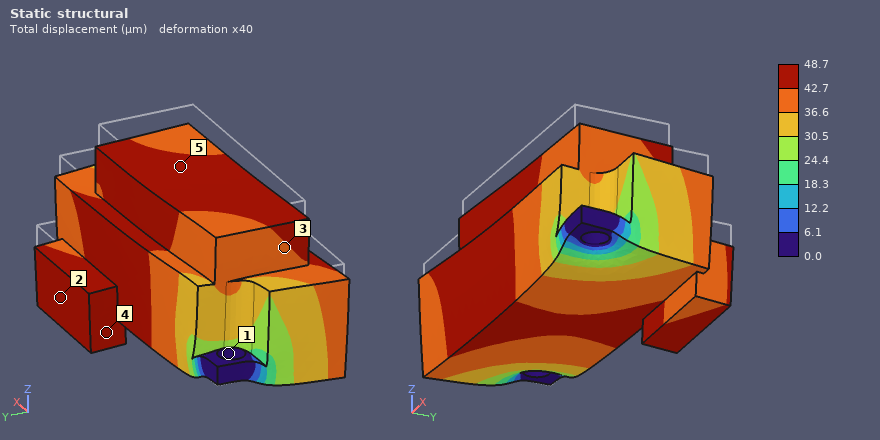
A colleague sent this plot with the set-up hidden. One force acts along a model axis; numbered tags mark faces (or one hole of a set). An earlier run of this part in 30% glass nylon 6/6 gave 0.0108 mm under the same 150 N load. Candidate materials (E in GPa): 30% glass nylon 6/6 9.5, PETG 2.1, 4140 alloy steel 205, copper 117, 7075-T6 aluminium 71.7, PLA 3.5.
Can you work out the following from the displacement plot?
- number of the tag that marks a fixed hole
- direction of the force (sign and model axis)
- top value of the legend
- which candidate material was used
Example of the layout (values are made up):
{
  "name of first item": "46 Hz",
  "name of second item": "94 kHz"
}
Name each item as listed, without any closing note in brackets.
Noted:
{
  "number of the tag that marks a fixed hole": "1",
  "direction of the force": "-Z",
  "top value of the legend": "48.7 µm",
  "which candidate material was used": "PETG"
}
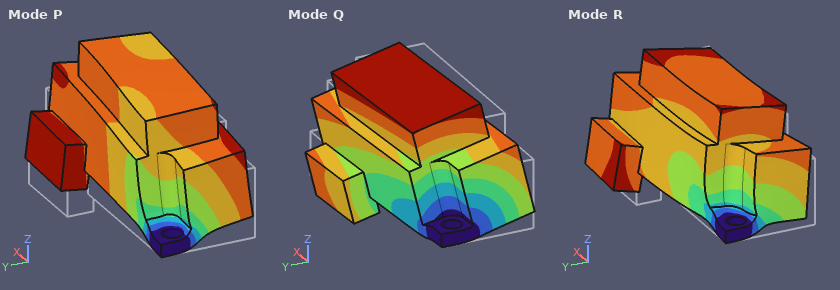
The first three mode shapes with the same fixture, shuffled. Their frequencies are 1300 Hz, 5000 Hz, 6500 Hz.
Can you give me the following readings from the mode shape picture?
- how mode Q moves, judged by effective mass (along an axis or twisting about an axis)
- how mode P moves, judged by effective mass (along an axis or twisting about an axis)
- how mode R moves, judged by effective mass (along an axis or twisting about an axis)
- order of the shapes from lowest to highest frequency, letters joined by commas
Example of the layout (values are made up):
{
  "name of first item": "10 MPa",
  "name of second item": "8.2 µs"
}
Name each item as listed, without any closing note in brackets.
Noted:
{
  "how mode Q moves, judged by effective mass": "along Y",
  "how mode P moves, judged by effective mass": "along Z",
  "how mode R moves, judged by effective mass": "along X",
  "order of the shapes from lowest to highest frequency, letters joined by commas": "Q, P, R"
}
